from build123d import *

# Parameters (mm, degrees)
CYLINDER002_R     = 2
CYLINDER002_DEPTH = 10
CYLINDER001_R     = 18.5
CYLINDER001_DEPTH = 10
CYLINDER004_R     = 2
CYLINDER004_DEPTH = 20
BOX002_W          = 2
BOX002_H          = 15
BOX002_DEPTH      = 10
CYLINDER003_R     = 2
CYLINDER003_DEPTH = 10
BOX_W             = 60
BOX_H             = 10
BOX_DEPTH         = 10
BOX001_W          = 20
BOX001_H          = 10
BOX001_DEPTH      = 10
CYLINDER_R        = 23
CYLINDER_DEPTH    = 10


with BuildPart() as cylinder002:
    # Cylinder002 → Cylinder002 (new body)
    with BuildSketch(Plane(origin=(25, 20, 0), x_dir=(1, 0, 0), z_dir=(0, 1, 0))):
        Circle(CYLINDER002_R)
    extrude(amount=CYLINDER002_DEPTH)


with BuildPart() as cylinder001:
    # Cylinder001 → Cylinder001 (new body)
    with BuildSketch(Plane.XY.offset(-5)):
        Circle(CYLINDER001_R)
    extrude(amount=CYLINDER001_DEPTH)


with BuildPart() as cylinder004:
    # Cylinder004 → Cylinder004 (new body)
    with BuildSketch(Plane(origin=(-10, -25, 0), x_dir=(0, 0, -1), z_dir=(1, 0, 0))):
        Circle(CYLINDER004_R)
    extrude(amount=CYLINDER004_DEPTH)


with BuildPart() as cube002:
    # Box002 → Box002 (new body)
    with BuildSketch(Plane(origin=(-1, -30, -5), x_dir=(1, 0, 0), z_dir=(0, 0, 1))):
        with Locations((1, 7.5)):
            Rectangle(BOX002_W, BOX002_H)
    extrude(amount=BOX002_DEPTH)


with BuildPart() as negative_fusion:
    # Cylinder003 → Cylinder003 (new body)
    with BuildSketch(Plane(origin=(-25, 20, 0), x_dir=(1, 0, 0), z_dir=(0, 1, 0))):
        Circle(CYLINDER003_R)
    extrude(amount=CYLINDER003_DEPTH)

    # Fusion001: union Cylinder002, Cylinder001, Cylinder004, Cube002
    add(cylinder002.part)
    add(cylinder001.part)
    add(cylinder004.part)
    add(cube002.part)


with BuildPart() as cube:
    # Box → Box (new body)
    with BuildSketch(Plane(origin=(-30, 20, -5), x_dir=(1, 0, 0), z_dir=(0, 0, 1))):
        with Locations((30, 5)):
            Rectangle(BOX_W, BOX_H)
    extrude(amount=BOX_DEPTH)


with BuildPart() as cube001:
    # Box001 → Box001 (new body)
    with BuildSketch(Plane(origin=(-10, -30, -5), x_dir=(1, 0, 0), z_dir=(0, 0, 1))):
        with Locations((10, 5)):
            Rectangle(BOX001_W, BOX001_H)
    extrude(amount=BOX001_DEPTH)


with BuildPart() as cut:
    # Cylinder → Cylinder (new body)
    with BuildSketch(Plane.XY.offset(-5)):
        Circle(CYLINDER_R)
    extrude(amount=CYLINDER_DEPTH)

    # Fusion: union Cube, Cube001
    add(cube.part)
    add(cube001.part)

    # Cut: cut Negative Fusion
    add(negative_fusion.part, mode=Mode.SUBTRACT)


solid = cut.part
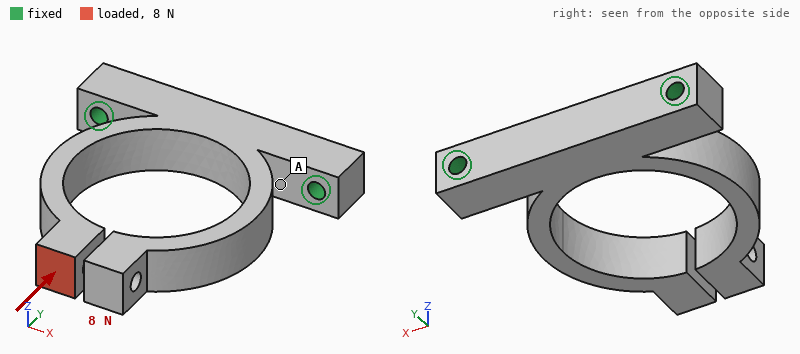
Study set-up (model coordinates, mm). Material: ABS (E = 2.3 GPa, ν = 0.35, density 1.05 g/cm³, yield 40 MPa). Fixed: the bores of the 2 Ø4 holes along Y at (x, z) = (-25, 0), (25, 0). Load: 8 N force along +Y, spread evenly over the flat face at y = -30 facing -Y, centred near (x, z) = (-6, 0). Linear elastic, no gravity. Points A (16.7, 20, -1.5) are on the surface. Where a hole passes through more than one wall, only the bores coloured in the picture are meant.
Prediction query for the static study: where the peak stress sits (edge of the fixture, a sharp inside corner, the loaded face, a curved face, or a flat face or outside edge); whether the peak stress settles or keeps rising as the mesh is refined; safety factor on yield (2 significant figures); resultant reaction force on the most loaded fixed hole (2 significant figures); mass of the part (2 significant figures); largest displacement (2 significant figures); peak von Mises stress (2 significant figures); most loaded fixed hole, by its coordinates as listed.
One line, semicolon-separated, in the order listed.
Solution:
a curved face; settles; 9.7; 5.4 N; 13 g; 0.83 mm; 4.1 MPa; (-25, 0)
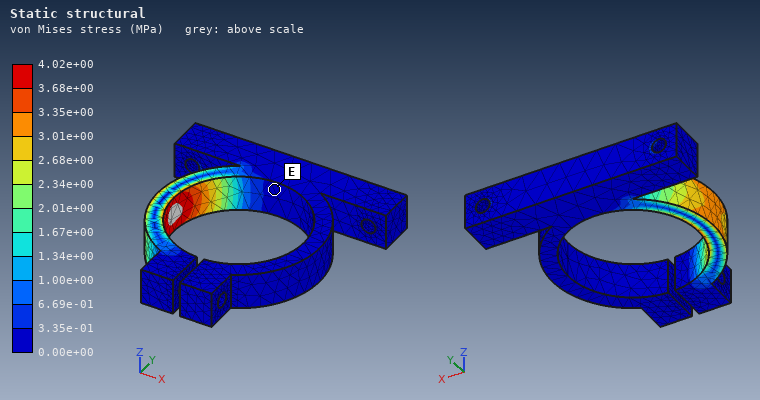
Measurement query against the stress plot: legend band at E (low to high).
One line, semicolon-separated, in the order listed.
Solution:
0.00e+00 to 3.35e-01 MPa
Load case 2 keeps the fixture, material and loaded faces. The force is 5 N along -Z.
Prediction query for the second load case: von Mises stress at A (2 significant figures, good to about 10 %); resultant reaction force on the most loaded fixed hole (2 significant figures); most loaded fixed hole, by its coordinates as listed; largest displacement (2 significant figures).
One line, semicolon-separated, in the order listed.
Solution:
0.81 MPa; 3.3 N; (-25, 0); 1.0 mm
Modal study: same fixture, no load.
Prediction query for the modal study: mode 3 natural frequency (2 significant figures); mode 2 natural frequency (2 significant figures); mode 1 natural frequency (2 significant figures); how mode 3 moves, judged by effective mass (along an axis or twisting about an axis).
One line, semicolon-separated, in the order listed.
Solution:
340 Hz; 280 Hz; 280 Hz; along Z
